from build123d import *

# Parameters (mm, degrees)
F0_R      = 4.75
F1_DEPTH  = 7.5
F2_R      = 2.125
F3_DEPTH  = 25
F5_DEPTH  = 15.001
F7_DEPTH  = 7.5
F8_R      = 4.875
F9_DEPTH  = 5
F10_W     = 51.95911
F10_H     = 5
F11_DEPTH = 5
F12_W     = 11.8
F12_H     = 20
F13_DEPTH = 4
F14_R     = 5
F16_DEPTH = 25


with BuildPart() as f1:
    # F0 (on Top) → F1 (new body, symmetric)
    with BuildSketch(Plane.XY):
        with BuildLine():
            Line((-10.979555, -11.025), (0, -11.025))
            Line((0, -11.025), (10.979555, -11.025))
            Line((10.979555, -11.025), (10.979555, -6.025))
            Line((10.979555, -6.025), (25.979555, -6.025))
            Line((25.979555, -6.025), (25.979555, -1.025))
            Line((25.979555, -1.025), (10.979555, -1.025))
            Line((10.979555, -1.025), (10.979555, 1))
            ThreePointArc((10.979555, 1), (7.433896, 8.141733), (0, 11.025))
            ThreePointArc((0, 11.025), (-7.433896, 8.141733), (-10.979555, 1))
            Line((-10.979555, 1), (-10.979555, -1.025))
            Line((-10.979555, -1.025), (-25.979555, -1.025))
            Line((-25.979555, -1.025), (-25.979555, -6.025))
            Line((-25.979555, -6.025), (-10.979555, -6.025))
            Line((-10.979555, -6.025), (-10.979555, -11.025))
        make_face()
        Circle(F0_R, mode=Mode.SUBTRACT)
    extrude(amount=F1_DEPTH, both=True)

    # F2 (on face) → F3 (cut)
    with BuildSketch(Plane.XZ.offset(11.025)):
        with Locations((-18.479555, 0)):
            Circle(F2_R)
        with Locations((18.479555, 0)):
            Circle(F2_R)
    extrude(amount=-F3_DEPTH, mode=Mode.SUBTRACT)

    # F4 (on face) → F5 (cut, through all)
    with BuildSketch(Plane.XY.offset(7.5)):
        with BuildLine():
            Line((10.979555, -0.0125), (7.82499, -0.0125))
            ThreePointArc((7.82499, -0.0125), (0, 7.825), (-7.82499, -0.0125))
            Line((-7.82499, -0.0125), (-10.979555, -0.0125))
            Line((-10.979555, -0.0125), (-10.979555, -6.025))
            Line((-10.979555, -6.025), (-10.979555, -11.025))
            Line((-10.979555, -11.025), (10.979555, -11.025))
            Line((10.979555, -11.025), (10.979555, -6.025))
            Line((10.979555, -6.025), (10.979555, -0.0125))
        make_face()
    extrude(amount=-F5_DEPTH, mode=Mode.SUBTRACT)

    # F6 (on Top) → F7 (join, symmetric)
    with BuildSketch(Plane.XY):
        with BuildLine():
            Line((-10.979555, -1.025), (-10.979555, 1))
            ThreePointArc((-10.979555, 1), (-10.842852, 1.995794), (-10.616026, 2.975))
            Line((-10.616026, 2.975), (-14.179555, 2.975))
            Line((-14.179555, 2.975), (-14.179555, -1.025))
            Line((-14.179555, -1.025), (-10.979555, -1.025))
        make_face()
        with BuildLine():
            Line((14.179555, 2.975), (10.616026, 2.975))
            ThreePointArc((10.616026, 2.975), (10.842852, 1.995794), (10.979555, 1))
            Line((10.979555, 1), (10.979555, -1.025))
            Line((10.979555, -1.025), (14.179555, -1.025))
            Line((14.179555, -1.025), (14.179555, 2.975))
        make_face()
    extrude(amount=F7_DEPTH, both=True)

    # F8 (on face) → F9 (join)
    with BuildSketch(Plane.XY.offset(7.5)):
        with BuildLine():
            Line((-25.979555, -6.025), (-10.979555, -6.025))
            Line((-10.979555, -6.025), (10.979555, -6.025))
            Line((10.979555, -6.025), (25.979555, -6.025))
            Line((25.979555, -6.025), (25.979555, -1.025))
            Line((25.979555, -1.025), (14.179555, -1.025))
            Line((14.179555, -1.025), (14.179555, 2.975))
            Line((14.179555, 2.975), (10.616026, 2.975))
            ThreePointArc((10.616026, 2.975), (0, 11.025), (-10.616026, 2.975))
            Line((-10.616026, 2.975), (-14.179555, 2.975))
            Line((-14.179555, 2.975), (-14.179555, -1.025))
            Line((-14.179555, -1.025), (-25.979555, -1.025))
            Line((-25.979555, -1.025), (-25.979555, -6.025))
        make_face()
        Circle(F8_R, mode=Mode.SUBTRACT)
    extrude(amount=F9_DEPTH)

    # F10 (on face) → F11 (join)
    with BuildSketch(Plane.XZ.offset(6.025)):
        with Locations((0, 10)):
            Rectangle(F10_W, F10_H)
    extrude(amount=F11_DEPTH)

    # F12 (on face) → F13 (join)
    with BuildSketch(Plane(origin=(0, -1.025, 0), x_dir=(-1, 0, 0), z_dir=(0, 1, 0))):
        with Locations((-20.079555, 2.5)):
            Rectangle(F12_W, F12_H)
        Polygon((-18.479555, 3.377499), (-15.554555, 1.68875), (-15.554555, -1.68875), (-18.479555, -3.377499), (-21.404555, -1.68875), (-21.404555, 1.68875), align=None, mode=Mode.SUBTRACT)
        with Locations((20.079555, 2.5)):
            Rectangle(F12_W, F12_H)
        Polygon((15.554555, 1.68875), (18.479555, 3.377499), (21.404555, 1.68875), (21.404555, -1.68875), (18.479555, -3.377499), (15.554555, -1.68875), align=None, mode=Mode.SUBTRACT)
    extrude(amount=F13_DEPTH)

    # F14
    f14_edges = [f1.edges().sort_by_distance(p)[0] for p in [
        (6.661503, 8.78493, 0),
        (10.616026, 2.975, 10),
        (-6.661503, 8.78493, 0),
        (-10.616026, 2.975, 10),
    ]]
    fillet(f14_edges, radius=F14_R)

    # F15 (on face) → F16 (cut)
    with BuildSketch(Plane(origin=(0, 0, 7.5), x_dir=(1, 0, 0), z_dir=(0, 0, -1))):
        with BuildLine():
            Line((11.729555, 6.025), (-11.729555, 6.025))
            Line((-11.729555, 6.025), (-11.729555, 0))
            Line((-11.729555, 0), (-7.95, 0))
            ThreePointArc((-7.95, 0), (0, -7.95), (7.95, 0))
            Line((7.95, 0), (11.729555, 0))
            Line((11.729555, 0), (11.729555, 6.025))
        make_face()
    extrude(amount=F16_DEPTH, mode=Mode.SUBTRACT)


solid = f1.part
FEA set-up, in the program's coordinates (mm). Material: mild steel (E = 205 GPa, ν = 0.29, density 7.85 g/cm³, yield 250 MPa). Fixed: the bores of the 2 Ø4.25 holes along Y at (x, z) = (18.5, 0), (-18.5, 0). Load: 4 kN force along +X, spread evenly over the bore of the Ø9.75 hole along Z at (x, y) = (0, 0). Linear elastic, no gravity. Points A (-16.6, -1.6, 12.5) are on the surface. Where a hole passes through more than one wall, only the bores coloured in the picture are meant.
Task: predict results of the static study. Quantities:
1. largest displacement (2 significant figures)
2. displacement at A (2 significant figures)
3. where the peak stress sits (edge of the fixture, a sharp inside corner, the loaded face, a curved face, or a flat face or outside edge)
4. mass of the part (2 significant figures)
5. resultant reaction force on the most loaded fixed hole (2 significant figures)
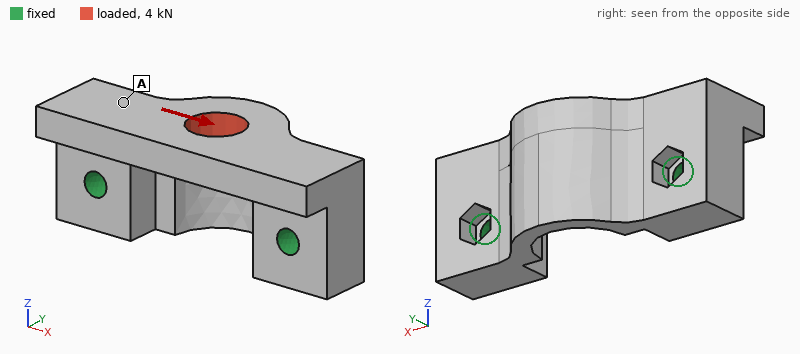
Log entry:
6.5 µm
5.2 µm
edge of the fixture
70 g
2.2 kN
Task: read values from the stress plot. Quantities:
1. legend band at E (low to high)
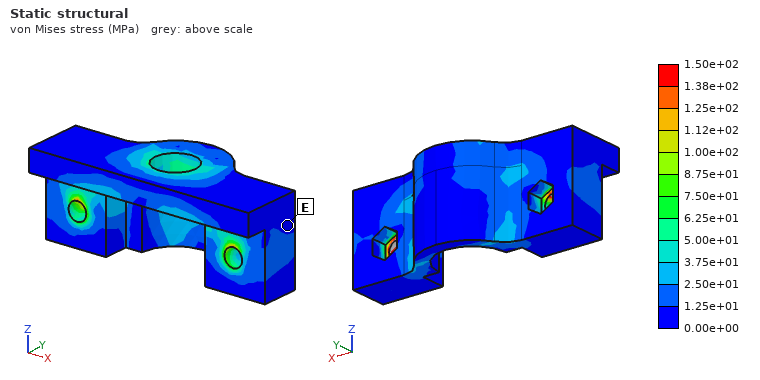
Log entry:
0.00e+00 to 1.25e+01 MPa
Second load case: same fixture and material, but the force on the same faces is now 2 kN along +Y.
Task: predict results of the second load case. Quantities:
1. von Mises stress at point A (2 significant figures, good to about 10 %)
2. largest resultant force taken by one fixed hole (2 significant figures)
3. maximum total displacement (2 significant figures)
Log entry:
21 MPa
1.0 kN
15 µm
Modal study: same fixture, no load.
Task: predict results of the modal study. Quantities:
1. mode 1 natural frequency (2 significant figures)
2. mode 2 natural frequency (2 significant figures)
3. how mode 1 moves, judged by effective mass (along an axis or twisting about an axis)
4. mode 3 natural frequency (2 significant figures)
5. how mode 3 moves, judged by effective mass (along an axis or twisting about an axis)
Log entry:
11 kHz
18 kHz
along Y
21 kHz
along Z
